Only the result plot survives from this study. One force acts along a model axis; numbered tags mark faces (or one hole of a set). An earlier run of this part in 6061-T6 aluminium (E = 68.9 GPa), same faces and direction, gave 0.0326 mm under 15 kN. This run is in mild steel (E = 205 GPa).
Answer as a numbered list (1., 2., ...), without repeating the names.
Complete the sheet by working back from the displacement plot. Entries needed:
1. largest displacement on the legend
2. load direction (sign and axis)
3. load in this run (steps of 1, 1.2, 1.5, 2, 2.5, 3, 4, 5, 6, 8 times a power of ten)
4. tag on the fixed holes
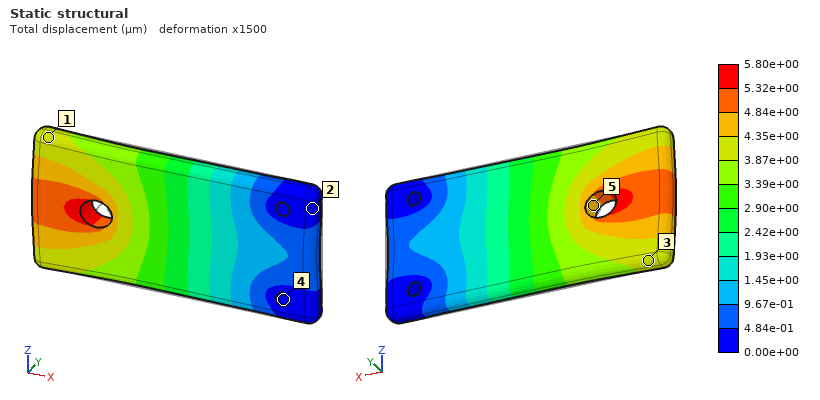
1. 5.80e+00 µm
2. -X
3. 8 kN
4. 4
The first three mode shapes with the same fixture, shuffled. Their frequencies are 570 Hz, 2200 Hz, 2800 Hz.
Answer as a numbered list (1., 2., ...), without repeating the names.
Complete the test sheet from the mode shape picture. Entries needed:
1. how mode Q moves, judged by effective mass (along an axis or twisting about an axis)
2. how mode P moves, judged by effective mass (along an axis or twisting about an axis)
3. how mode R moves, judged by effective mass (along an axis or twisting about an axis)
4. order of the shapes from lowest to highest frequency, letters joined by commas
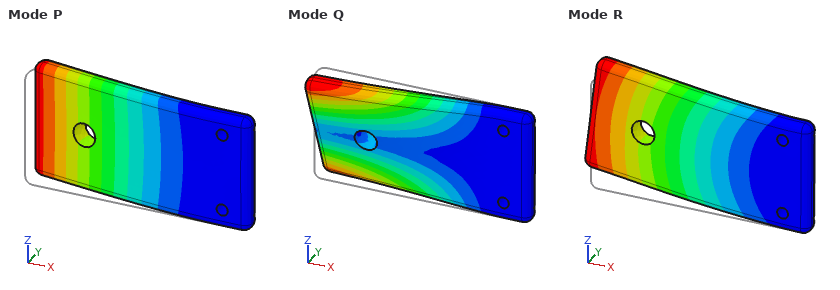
1. twisting about X
2. along Y
3. along Z
4. P, Q, R
